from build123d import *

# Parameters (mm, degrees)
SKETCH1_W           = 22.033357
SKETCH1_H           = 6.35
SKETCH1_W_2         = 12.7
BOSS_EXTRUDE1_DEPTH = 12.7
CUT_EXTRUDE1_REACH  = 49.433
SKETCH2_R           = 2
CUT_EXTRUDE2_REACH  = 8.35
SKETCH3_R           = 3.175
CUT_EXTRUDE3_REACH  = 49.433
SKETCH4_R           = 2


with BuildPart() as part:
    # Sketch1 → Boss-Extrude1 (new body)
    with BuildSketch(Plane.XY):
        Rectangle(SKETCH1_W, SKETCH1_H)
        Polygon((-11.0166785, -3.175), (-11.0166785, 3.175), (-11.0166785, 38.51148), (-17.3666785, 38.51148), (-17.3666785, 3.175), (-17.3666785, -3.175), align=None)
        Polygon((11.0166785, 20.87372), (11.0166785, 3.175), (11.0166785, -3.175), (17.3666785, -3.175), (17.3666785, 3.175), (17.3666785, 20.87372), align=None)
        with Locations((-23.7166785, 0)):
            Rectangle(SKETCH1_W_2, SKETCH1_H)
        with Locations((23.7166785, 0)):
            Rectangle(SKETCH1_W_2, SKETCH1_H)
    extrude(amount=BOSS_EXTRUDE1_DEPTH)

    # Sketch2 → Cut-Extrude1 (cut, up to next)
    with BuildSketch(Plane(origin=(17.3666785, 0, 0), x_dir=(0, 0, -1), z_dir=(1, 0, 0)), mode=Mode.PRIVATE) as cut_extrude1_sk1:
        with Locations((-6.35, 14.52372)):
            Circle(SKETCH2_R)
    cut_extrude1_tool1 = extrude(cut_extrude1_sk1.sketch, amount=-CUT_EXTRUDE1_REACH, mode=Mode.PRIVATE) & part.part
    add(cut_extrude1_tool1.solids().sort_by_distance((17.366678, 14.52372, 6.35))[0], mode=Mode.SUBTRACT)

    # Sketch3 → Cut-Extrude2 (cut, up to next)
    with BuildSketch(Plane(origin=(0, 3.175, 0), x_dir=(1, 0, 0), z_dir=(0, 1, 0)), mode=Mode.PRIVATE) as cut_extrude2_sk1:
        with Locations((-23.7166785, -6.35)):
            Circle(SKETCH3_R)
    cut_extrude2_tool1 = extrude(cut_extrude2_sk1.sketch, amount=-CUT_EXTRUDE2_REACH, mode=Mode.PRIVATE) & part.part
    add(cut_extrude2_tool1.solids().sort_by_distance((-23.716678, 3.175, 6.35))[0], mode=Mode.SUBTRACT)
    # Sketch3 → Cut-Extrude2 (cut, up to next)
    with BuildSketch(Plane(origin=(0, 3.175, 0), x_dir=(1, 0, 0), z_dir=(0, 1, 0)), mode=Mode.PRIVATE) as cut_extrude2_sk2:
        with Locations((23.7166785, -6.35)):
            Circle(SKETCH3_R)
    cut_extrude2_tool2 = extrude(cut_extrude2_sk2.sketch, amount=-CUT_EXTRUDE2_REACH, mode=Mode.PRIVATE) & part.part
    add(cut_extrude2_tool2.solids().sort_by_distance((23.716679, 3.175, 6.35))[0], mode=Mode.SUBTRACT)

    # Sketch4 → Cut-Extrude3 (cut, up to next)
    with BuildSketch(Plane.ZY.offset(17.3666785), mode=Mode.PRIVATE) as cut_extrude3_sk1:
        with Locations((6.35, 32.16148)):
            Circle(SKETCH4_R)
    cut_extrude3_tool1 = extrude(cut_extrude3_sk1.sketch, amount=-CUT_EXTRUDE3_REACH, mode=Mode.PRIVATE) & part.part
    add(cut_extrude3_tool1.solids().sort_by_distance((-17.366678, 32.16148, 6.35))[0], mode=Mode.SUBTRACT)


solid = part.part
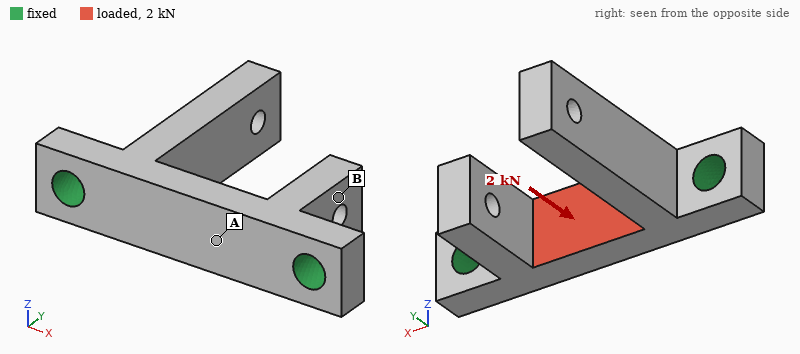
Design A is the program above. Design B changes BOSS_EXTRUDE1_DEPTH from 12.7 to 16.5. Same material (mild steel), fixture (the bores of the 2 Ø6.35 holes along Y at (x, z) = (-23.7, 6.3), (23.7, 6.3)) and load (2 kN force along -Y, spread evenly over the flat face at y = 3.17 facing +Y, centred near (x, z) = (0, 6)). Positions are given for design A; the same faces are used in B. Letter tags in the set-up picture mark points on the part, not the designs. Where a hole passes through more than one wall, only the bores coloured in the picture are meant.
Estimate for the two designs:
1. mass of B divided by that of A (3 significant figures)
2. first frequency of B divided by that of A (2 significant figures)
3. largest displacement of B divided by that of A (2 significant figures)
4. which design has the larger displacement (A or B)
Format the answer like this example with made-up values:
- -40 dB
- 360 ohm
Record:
- 1.32
- 0.99
- 0.84
- A
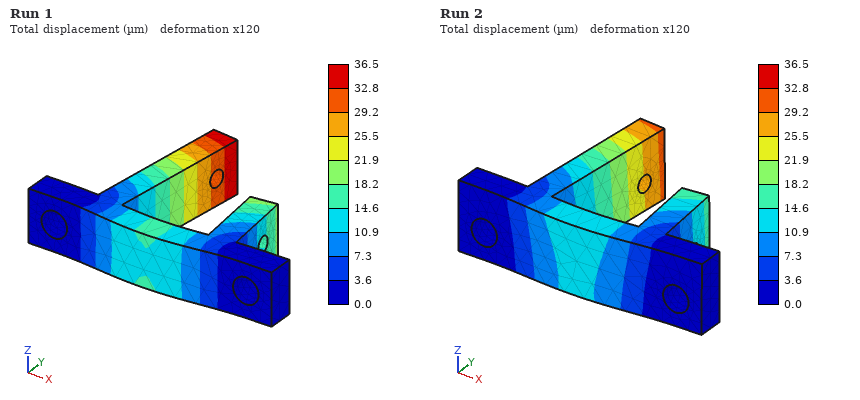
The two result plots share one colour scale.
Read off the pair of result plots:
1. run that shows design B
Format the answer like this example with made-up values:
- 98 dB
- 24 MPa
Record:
- Run 2
